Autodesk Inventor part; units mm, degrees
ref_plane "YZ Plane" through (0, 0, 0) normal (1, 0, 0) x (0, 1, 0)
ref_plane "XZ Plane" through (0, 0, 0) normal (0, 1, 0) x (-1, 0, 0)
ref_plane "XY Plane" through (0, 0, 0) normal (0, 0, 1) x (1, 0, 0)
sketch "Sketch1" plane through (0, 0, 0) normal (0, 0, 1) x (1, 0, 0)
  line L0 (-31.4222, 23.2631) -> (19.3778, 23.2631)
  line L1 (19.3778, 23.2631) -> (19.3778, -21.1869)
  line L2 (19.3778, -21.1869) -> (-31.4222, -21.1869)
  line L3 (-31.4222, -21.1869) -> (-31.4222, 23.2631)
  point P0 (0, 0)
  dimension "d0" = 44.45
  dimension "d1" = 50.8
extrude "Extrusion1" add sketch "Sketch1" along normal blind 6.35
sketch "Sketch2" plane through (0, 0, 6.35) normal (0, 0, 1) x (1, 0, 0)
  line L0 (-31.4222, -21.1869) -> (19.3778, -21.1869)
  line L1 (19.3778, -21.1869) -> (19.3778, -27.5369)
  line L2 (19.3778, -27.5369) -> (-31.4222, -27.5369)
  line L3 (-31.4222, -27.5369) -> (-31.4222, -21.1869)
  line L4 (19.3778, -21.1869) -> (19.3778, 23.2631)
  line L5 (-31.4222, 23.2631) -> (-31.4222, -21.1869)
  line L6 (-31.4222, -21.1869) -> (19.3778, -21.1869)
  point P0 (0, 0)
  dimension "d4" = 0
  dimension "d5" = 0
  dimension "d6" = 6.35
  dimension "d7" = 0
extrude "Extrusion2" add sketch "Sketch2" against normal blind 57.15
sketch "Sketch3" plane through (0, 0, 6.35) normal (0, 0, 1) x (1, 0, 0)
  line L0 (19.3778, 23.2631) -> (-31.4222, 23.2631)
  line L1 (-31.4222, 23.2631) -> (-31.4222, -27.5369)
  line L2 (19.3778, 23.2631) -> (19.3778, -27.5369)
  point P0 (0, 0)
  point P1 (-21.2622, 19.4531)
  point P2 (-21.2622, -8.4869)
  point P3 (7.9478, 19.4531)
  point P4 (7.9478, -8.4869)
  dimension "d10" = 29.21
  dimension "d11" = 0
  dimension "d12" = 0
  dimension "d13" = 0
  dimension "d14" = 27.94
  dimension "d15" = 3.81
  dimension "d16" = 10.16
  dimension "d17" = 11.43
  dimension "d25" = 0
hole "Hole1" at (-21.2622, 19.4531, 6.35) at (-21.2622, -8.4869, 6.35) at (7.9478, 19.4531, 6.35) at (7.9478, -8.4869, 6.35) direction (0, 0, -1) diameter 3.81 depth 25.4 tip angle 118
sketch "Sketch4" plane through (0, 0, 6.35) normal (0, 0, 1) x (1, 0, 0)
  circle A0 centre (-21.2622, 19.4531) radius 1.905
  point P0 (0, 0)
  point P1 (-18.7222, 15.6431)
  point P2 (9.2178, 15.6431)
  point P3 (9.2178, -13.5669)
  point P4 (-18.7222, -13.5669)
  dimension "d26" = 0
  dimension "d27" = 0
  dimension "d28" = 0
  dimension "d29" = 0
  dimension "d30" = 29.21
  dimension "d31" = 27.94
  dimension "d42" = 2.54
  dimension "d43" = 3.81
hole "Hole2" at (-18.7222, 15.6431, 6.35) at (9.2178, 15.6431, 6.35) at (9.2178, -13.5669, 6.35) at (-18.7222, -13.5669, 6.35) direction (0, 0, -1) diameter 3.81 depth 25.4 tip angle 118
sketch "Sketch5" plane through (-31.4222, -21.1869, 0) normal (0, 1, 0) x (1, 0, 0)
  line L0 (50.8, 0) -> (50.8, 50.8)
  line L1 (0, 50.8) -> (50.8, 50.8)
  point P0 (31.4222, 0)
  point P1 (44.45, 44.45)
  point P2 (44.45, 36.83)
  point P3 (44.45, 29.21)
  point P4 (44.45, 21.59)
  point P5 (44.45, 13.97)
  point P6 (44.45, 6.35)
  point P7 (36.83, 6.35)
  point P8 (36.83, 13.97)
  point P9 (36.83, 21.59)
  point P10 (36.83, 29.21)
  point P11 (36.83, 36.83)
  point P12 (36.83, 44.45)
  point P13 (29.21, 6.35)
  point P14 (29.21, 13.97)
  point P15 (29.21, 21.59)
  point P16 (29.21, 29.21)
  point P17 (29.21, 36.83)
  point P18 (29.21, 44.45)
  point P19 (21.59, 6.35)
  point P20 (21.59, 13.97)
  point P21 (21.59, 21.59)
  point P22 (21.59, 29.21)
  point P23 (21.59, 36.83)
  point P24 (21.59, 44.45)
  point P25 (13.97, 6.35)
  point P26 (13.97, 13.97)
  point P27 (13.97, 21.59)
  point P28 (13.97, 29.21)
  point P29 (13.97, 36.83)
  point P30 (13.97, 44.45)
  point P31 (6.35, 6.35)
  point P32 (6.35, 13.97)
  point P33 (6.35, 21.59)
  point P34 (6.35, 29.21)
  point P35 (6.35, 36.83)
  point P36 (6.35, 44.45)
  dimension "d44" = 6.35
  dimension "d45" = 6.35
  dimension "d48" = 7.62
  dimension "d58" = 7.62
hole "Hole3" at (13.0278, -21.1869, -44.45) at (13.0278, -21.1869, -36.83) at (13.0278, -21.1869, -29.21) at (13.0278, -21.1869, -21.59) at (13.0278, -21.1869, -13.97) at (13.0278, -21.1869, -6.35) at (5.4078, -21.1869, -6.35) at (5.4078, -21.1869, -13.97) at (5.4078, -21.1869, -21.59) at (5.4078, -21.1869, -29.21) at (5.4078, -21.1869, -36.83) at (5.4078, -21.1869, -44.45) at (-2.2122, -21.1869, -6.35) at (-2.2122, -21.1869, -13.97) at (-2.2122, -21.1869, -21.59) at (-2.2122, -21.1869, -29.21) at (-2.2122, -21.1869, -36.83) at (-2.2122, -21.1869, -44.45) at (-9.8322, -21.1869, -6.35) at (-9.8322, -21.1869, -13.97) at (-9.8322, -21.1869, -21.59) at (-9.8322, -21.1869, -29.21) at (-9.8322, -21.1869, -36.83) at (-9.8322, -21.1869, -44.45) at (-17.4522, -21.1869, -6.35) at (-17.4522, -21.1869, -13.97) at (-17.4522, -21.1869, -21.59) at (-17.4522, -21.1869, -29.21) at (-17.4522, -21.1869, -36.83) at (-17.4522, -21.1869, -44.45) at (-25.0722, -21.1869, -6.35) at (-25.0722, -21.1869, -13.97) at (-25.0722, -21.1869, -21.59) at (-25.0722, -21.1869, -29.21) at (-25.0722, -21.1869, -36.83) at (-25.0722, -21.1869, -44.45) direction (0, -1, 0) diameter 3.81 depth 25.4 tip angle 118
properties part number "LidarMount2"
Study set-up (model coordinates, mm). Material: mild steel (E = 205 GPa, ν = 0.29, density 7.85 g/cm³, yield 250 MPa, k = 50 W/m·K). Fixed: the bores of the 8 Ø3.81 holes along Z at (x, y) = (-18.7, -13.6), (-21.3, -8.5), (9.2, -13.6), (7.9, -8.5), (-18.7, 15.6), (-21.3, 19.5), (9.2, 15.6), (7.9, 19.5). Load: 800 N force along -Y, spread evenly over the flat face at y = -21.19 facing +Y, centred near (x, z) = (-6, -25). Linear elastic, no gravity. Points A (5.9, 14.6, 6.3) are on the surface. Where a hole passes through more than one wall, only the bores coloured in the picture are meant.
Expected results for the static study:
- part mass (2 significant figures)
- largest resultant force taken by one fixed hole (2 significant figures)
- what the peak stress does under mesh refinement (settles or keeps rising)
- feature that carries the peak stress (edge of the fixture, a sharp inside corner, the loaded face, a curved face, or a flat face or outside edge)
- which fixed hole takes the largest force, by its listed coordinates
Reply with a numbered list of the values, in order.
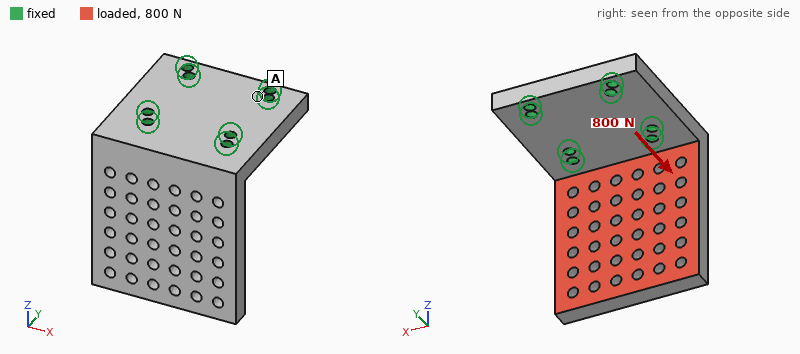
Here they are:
1. 230 g
2. 620 N
3. keeps rising
4. edge of the fixture
5. (-18.7, -13.6)
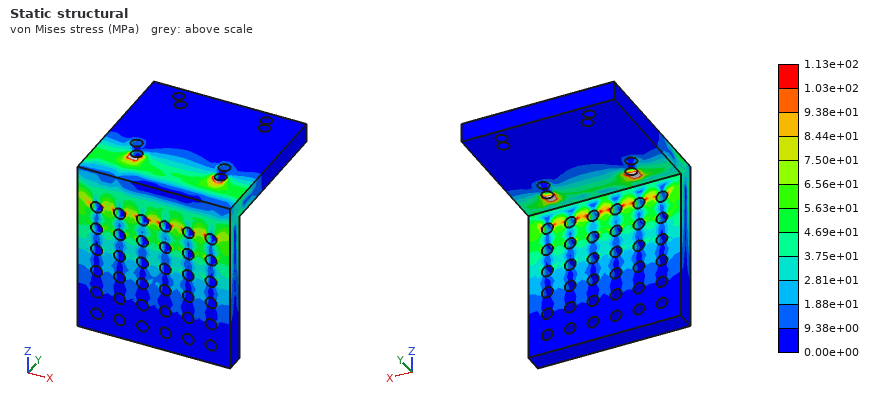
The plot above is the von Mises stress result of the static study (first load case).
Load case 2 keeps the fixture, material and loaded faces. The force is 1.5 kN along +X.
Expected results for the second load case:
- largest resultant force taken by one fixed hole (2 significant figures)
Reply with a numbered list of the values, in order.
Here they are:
1. 1.6 kN
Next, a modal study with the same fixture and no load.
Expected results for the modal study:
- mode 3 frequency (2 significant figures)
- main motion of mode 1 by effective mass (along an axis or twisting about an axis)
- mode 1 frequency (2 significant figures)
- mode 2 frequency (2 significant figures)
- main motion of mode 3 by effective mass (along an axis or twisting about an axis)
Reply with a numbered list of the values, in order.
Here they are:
1. 4600 Hz
2. along Y
3. 1400 Hz
4. 3400 Hz
5. along X
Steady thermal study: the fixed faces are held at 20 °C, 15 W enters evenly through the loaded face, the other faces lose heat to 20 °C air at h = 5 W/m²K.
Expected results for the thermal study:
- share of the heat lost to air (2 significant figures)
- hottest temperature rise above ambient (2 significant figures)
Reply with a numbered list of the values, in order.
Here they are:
1. 6.7 %
2. 42 K
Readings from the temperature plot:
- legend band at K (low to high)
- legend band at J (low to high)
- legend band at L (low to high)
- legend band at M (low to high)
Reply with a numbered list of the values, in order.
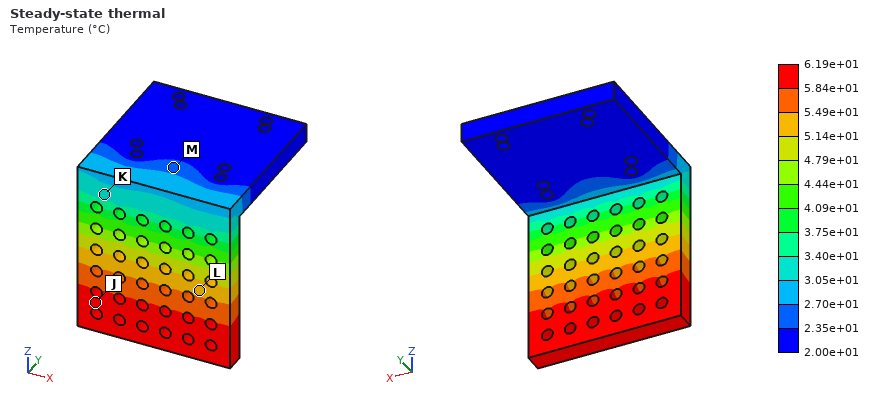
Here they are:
1. 3.05e+01 to 3.40e+01 °C
2. 5.84e+01 to 6.19e+01 °C
3. 5.14e+01 to 5.49e+01 °C
4. 2.35e+01 to 2.70e+01 °C
